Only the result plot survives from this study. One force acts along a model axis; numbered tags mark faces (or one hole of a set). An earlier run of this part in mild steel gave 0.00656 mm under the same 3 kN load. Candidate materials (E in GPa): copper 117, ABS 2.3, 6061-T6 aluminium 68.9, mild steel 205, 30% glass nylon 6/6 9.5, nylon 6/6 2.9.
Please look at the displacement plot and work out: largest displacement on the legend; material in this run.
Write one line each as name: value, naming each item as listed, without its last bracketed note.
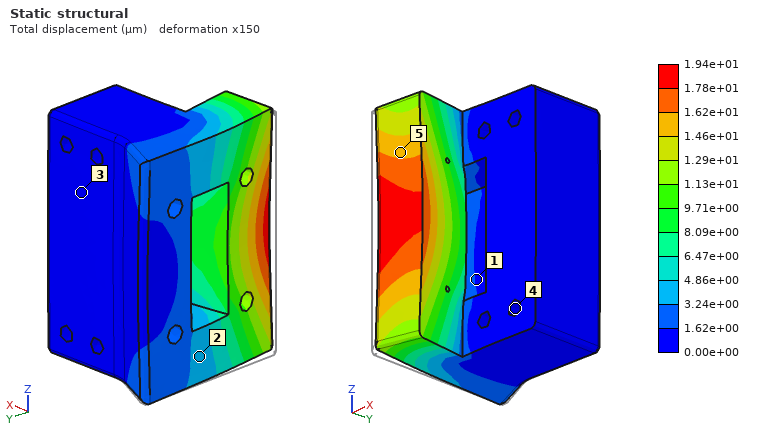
largest displacement on the legend: 1.94e+01 µm
material in this run: 6061-T6 aluminium
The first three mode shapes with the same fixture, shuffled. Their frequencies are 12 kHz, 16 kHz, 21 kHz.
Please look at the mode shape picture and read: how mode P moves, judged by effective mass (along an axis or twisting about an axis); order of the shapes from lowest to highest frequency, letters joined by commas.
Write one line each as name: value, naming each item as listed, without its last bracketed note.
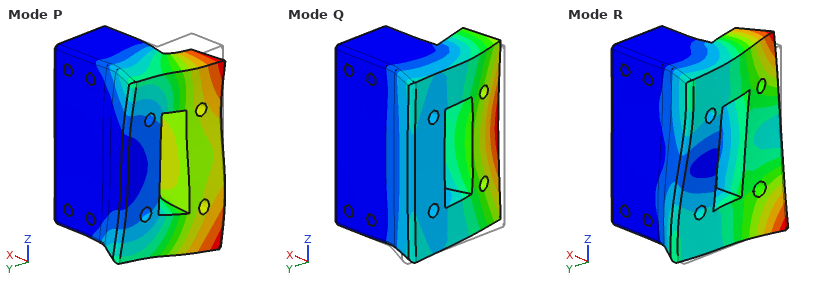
how mode P moves, judged by effective mass: along Z
order of the shapes from lowest to highest frequency, letters joined by commas: Q, P, R
